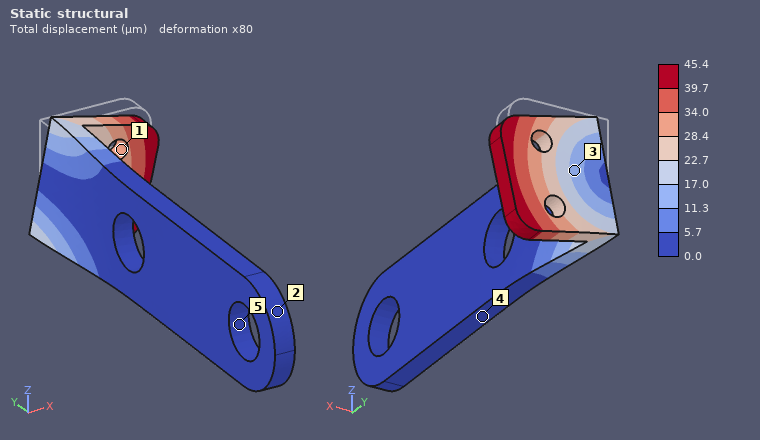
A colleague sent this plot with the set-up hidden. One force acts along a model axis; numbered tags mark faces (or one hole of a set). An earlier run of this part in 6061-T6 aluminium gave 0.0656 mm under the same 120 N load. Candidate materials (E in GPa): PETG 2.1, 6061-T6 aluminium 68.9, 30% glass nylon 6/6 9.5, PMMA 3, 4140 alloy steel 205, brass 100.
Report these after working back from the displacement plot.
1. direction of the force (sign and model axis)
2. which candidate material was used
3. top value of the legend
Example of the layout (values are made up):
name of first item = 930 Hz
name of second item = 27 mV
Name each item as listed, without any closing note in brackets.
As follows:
direction of the force = -Z
which candidate material was used = brass
top value of the legend = 45.4 µm
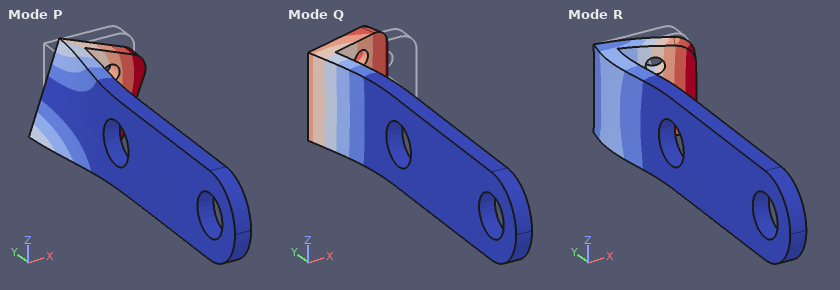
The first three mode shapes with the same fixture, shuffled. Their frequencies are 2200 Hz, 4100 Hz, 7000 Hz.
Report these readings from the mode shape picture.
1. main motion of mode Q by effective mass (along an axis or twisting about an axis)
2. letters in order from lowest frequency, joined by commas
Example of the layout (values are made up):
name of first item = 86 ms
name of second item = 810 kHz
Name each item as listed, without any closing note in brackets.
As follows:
main motion of mode Q by effective mass = along X
letters in order from lowest frequency, joined by commas = Q, P, R
